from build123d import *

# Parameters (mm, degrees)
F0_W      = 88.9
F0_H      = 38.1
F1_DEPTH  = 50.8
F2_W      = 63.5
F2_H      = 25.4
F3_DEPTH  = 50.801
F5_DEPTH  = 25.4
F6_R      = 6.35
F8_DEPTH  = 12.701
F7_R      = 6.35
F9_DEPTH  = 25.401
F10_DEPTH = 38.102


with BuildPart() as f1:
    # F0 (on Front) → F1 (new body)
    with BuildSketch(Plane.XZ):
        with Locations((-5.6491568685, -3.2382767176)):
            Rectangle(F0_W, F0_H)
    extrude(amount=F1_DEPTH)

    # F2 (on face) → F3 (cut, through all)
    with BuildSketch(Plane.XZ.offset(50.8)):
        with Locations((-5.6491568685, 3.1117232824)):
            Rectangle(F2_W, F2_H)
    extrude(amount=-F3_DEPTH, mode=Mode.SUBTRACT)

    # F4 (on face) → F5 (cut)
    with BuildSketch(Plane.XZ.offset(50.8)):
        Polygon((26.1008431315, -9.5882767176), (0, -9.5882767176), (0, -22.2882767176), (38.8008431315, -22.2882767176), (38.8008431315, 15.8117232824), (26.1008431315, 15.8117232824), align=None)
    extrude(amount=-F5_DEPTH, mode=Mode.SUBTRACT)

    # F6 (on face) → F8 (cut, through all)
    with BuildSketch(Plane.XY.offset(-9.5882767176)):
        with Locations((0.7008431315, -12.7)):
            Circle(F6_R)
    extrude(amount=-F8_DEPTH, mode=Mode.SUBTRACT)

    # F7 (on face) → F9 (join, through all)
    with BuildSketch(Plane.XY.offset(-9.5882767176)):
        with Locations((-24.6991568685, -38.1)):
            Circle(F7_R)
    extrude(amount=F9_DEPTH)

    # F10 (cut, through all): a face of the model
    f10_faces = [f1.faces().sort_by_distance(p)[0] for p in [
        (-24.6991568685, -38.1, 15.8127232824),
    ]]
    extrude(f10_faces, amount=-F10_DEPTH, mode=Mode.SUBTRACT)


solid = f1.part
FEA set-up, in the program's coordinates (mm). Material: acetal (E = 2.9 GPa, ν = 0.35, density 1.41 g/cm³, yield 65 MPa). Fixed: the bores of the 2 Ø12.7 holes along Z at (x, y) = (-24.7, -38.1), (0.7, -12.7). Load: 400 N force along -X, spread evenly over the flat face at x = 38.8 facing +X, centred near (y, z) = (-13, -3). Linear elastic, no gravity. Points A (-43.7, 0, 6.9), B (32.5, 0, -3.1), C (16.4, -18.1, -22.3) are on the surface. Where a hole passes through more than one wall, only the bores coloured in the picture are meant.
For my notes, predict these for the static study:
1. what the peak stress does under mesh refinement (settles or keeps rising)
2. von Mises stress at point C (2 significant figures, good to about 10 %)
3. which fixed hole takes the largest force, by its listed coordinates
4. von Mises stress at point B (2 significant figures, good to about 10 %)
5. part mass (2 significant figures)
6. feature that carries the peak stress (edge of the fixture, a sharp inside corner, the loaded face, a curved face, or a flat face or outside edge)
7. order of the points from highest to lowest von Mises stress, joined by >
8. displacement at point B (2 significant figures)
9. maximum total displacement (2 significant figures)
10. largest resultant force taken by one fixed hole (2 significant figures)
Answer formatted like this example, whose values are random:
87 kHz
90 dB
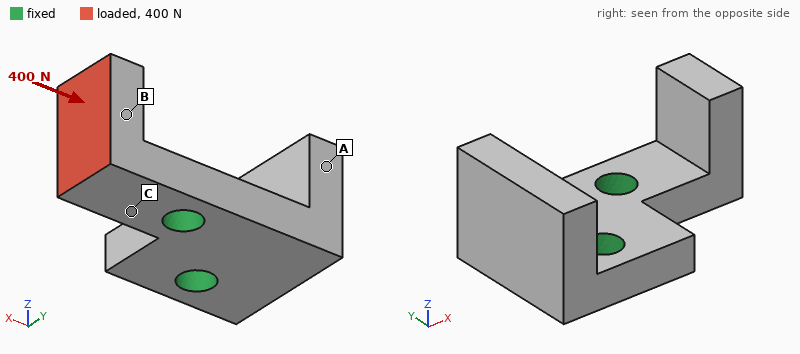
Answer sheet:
keeps rising
6.0 MPa
(0.7, -12.7)
2.0 MPa
93 g
edge of the fixture
C > B > A
0.22 mm
0.48 mm
390 N
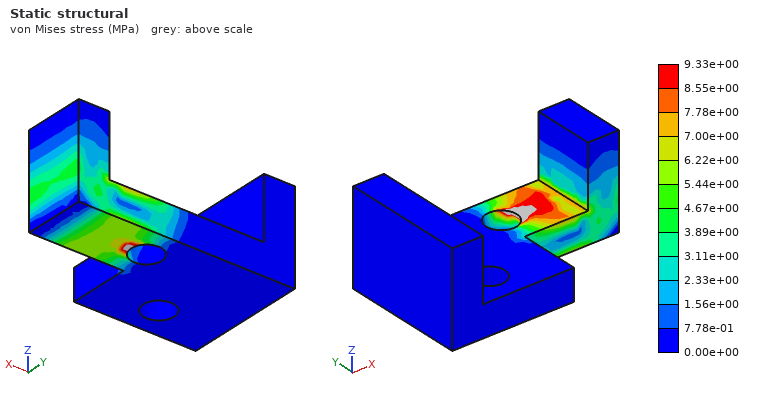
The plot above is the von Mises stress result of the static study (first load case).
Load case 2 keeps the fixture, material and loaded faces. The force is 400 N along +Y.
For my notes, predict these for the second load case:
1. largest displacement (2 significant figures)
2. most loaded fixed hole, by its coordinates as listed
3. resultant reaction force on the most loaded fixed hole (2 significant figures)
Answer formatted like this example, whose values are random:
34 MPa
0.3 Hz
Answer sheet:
0.50 mm
(0.7, -12.7)
450 N
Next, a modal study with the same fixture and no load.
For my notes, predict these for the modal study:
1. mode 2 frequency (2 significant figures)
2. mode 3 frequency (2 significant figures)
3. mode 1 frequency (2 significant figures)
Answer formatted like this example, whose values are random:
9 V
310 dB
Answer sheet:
1300 Hz
1300 Hz
1100 Hz
